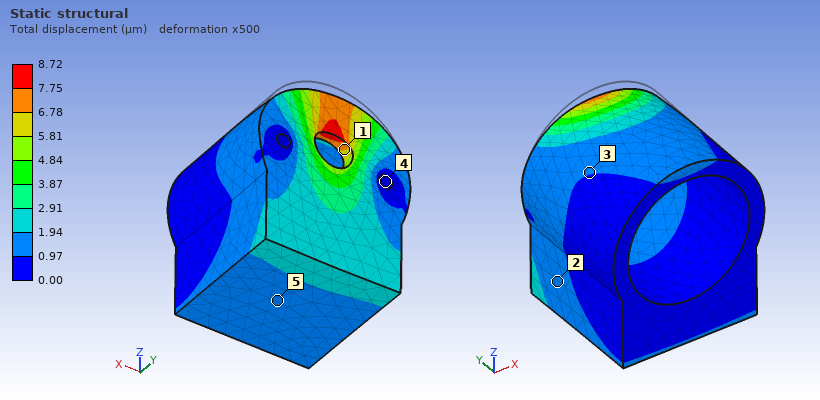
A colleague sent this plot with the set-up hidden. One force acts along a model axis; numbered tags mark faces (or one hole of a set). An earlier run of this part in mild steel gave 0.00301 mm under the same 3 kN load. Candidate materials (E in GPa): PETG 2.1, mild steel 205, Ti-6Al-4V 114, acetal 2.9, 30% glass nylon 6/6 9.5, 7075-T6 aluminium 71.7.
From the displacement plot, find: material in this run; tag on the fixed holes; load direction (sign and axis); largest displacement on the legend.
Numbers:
7075-T6 aluminium
4
-Z
8.72 µm
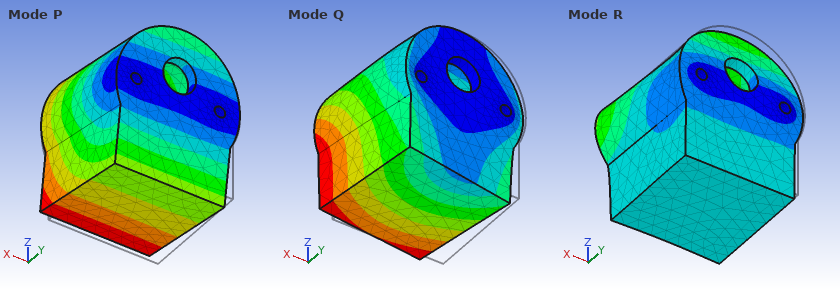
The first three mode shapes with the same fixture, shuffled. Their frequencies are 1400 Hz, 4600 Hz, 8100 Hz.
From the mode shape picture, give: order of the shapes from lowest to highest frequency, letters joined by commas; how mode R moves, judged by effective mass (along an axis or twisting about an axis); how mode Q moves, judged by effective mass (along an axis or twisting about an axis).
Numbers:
P, Q, R
along Y
along X
